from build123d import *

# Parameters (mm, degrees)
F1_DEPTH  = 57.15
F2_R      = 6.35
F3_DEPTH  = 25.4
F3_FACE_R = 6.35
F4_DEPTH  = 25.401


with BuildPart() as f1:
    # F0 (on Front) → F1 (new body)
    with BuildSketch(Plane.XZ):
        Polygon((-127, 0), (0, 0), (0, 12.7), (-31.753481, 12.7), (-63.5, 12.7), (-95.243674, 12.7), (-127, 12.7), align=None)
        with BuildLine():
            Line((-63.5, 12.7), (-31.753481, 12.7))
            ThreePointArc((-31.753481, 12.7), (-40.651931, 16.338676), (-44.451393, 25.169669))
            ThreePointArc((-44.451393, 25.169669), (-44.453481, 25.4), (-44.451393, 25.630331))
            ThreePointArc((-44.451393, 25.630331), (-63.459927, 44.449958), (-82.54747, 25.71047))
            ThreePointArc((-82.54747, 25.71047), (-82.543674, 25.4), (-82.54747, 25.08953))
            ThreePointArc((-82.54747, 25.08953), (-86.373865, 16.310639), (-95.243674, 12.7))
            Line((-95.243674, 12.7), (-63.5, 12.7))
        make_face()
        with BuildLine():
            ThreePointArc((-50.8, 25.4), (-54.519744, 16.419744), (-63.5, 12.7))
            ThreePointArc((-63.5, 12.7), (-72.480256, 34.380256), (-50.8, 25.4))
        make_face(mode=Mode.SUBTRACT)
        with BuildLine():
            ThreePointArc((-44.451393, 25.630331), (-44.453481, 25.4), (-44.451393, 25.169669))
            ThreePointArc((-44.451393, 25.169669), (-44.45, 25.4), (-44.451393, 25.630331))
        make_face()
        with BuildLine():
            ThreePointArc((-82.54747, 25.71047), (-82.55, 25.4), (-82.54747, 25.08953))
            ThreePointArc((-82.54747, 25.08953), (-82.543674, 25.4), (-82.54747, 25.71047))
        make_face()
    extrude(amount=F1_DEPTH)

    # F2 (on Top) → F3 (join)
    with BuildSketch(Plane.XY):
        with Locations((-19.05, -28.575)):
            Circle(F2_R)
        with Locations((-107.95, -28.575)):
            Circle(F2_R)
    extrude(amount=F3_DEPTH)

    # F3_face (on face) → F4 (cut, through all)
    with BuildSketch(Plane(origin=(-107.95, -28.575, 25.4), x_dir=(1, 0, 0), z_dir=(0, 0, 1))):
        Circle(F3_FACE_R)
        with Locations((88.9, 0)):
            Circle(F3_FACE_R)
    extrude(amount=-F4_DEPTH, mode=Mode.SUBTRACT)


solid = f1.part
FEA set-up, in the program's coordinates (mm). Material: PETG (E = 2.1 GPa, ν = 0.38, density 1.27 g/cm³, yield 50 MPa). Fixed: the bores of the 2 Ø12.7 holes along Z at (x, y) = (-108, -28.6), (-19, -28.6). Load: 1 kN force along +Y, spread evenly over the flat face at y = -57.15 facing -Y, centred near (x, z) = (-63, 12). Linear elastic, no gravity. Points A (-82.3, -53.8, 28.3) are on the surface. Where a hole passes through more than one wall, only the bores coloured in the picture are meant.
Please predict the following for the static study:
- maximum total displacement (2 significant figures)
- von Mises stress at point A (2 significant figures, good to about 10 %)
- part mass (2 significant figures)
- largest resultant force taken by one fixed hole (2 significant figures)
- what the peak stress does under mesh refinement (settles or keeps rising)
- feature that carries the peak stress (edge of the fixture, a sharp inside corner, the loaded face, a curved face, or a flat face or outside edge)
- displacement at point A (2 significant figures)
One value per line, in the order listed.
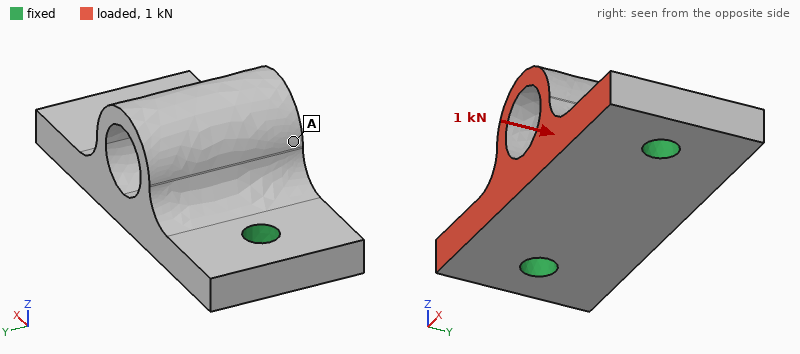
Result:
0.12 mm
0.53 MPa
160 g
500 N
keeps rising
edge of the fixture
0.087 mm
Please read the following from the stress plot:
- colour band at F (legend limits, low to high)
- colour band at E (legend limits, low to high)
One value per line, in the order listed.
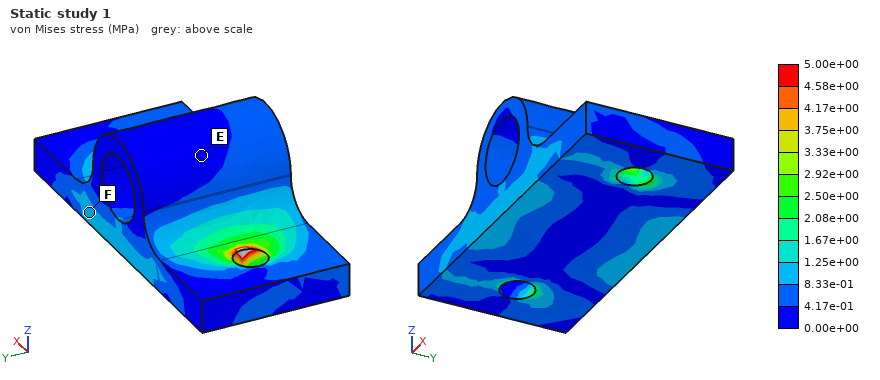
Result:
8.33e-01 to 1.25e+00 MPa
0.00e+00 to 4.17e-01 MPa
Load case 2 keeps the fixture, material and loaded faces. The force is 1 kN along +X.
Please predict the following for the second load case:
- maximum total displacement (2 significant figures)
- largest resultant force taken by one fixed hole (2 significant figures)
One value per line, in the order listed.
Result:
83 µm
580 N
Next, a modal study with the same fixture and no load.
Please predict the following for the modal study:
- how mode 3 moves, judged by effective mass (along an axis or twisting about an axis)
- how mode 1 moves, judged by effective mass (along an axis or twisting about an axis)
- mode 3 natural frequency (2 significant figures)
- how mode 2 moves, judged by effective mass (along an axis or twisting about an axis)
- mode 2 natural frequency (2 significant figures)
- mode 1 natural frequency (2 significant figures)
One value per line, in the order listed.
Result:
along X
along Y
2500 Hz
along Z
1700 Hz
1200 Hz
